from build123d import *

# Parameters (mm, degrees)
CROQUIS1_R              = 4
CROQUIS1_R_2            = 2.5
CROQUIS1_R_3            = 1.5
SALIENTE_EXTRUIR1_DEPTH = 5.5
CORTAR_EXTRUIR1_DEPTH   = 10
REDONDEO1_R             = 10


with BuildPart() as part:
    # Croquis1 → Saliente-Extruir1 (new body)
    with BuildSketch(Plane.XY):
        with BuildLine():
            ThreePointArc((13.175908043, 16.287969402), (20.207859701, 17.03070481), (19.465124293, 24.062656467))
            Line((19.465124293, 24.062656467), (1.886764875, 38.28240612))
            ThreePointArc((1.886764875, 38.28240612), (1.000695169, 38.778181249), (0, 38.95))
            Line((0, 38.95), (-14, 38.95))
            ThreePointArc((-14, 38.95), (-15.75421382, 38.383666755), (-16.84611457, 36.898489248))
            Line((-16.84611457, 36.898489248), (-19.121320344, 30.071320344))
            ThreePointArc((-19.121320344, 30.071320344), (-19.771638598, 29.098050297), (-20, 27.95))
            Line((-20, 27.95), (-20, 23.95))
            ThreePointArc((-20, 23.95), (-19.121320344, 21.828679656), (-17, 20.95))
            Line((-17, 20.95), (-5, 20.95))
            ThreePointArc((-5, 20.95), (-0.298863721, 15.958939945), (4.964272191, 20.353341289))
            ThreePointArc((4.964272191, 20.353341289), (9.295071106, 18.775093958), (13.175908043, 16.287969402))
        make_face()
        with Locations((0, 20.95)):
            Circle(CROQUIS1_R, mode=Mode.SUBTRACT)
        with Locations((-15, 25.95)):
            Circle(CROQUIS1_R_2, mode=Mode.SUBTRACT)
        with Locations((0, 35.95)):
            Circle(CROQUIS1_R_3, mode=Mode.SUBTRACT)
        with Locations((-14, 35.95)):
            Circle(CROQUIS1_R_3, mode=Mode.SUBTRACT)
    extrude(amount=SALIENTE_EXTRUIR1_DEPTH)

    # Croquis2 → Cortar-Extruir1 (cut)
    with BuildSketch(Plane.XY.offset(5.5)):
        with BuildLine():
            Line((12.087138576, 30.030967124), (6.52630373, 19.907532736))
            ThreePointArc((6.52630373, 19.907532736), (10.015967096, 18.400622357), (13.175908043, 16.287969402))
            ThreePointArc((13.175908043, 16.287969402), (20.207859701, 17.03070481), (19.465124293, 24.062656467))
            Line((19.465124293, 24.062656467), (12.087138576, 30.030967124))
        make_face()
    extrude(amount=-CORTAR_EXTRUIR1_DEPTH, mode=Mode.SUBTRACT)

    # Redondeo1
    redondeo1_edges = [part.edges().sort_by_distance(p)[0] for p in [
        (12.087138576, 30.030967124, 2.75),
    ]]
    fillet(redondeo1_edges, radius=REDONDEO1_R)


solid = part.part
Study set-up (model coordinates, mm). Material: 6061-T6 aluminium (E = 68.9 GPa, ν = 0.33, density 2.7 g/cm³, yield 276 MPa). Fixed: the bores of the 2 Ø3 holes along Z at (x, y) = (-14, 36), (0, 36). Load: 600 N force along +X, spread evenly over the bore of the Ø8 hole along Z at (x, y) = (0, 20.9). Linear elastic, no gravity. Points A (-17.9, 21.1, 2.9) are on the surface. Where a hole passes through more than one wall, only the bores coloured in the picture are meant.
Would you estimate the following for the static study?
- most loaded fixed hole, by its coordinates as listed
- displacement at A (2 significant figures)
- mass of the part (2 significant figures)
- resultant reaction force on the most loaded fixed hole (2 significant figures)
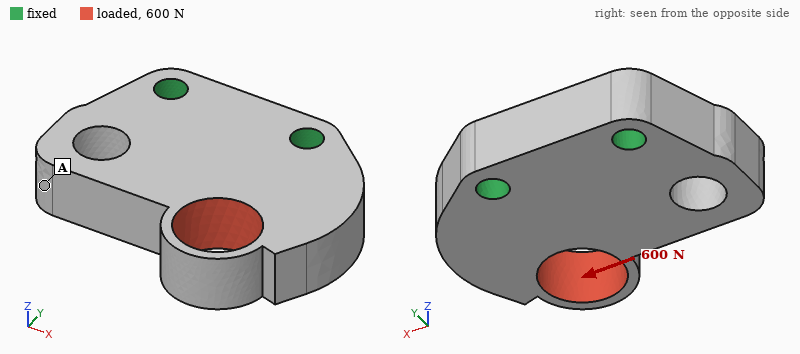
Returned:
(-14, 36)
4.9 µm
6.3 g
670 N
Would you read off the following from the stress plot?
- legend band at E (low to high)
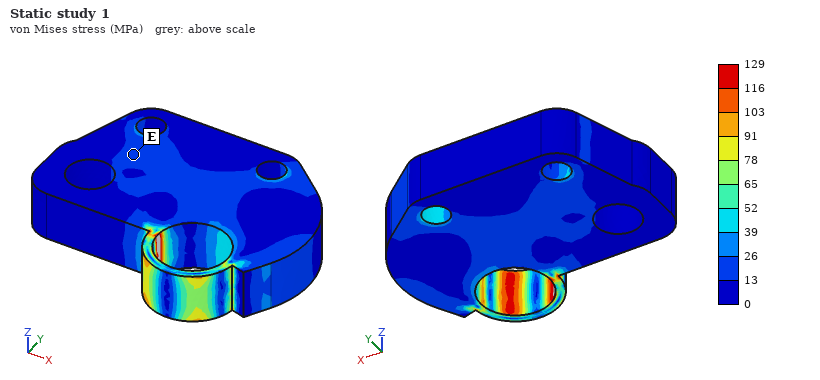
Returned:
13 to 26 MPa
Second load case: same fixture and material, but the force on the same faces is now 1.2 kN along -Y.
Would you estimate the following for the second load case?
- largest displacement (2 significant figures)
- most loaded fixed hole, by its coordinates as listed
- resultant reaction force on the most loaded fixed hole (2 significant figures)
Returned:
17 µm
(0, 36)
1.1 kN
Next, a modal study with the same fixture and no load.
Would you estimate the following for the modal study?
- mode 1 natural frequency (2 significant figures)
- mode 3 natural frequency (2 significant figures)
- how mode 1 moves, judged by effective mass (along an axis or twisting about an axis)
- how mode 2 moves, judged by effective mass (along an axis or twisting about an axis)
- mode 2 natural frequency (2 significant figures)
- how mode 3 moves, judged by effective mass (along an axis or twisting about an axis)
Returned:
16 kHz
29 kHz
along Z
twisting about Y
23 kHz
along X
